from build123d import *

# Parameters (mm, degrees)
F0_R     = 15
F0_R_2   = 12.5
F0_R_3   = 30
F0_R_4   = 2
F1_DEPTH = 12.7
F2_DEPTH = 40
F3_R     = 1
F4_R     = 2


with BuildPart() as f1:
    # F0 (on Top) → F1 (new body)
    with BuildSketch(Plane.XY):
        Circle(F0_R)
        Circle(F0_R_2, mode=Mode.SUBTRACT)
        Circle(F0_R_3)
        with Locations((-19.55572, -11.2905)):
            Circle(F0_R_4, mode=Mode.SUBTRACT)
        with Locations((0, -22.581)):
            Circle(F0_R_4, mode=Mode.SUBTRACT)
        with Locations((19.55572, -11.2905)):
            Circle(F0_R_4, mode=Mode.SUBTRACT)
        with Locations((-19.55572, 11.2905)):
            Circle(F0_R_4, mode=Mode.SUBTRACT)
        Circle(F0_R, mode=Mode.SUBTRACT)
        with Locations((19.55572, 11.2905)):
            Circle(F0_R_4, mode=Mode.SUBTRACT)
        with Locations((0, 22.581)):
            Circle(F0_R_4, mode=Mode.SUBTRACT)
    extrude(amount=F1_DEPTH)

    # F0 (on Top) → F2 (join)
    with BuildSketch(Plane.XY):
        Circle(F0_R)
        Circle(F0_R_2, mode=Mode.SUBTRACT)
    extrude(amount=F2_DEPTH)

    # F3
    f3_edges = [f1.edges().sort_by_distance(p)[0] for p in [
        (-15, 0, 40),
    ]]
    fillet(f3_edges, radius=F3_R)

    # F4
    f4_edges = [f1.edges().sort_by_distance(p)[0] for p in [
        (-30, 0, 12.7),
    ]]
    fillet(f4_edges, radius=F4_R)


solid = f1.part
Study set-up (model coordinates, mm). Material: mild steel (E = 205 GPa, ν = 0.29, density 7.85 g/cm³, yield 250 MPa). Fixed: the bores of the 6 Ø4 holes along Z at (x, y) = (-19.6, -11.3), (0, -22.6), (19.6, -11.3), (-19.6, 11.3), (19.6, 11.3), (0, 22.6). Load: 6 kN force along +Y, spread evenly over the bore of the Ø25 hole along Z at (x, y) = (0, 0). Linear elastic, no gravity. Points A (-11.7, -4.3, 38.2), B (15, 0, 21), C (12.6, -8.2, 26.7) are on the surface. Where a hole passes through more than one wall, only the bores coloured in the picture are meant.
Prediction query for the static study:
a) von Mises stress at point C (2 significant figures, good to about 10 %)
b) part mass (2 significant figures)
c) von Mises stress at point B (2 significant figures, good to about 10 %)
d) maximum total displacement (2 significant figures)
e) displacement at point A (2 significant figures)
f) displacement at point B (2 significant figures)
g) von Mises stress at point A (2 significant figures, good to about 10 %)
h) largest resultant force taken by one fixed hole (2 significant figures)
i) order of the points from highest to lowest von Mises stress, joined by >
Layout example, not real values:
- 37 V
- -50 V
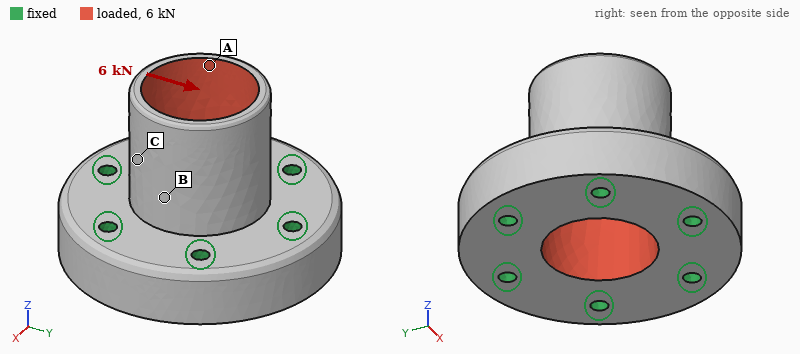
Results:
- 26 MPa
- 270 g
- 39 MPa
- 13 µm
- 12 µm
- 4.9 µm
- 7.8 MPa
- 1.8 kN
- B > C > A
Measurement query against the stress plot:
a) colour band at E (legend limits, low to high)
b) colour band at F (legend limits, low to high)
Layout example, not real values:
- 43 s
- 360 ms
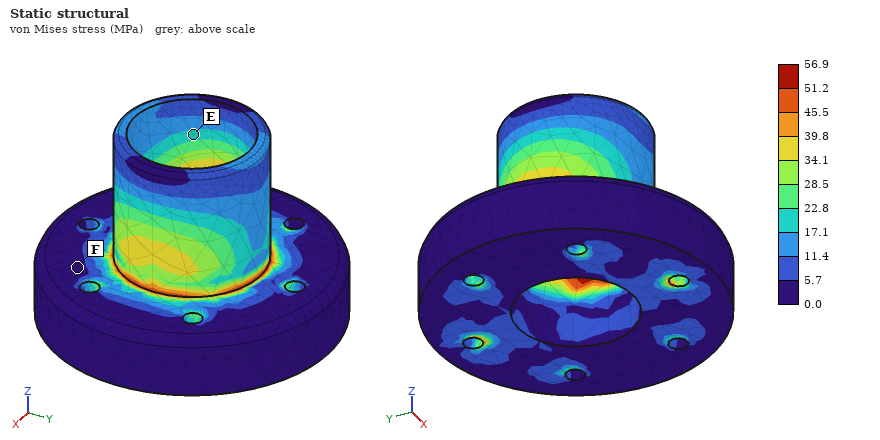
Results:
- 17.1 to 22.8 MPa
- 0.0 to 5.7 MPa
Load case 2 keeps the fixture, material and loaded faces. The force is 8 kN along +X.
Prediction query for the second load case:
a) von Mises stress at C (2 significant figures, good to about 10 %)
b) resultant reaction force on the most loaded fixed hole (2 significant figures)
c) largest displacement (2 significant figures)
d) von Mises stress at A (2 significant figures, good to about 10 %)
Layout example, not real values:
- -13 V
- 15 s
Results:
- 27 MPa
- 2.2 kN
- 17 µm
- 16 MPa
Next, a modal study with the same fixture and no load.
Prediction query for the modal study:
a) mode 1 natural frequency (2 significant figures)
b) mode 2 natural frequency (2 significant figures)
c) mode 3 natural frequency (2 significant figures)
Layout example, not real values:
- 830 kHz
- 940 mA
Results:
- 12 kHz
- 12 kHz
- 15 kHz
